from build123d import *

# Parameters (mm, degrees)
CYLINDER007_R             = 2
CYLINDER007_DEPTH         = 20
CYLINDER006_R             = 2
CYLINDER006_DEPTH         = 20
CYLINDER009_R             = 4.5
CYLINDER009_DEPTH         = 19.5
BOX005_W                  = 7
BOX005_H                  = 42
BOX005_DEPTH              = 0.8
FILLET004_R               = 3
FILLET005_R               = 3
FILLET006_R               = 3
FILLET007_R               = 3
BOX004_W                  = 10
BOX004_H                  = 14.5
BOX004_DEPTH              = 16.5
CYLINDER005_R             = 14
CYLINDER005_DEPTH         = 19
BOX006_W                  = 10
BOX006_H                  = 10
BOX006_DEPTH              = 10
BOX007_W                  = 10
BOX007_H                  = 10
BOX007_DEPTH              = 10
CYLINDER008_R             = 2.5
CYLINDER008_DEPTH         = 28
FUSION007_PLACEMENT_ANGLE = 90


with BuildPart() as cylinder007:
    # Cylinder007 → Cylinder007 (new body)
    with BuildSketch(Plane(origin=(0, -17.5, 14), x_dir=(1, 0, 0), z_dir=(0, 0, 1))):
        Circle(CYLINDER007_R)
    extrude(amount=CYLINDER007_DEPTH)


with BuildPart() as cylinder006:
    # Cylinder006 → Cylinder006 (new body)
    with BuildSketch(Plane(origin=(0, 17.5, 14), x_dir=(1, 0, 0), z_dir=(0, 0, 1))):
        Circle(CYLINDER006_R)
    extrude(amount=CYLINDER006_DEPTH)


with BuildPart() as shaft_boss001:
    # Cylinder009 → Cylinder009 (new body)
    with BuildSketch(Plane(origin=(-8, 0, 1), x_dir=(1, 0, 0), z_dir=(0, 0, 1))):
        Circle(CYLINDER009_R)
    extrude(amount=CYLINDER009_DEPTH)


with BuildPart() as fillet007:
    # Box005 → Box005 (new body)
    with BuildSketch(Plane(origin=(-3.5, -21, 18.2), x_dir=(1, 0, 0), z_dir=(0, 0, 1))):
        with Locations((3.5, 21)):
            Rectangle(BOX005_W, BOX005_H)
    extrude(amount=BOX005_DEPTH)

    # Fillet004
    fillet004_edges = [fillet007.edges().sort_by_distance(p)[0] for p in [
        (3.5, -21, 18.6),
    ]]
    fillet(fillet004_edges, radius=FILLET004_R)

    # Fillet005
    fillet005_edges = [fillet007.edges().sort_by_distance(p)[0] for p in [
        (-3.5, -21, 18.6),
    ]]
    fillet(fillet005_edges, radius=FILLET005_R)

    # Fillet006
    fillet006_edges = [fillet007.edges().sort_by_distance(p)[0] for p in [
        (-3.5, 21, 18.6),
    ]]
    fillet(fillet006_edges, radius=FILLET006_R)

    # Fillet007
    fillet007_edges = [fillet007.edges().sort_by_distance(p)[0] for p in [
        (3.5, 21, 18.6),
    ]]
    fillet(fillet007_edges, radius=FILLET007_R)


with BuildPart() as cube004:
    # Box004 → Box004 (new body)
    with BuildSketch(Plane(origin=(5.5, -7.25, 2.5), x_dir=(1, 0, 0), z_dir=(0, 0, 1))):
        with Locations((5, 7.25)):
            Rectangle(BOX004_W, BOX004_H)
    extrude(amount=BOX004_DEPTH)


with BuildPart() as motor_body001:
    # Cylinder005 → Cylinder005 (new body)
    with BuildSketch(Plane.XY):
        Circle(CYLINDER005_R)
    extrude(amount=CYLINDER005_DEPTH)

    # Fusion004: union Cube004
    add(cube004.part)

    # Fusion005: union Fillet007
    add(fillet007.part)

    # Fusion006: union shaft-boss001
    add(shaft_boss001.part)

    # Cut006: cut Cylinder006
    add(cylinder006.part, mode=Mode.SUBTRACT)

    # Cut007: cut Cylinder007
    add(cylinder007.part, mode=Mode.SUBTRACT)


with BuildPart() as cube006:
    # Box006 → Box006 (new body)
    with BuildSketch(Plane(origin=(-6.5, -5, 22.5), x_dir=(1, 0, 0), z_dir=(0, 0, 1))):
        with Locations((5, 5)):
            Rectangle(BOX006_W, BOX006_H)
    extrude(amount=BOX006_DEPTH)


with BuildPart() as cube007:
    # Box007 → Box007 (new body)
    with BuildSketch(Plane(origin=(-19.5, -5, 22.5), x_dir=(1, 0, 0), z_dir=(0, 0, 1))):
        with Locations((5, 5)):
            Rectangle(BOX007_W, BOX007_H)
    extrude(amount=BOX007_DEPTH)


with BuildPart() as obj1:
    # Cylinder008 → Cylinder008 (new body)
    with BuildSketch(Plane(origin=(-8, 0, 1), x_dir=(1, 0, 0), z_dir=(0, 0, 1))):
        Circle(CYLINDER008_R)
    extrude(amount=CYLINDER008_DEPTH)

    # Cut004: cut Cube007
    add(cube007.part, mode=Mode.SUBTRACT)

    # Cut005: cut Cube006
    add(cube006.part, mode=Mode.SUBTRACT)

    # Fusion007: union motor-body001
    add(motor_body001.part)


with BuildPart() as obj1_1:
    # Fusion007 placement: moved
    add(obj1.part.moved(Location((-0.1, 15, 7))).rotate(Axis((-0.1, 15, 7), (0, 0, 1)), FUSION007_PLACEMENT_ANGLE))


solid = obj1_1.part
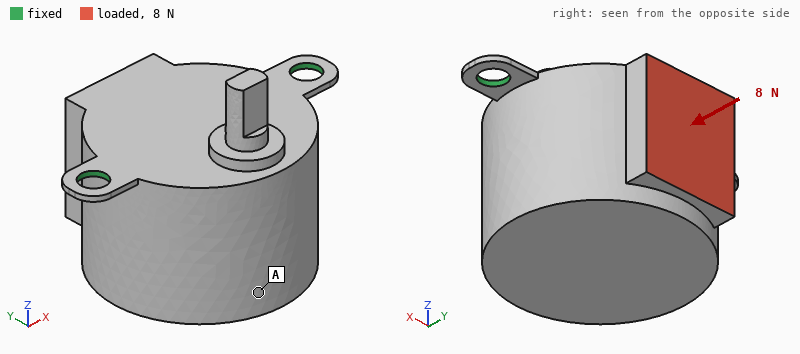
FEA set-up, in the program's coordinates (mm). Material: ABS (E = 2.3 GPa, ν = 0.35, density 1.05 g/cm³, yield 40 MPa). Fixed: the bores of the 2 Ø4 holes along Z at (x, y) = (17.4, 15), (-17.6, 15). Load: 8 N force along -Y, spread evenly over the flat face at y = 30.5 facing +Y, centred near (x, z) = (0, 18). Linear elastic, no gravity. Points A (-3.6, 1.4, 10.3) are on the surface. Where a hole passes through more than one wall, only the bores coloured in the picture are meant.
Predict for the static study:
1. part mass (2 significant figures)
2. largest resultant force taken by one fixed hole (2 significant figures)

13 g
4.0 N
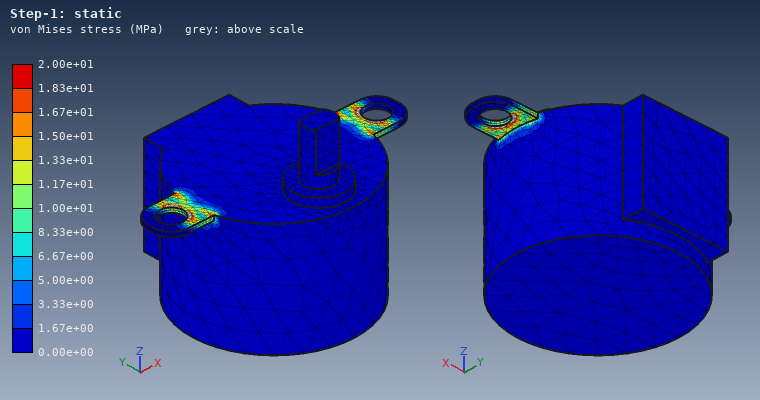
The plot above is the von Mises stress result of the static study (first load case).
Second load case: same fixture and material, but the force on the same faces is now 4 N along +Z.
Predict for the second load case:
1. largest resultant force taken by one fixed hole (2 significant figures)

2.4 N
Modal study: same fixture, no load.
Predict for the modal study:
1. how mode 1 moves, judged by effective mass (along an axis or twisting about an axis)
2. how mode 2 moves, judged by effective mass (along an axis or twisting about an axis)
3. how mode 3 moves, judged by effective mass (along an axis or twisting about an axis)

along Y
along Z
along X
